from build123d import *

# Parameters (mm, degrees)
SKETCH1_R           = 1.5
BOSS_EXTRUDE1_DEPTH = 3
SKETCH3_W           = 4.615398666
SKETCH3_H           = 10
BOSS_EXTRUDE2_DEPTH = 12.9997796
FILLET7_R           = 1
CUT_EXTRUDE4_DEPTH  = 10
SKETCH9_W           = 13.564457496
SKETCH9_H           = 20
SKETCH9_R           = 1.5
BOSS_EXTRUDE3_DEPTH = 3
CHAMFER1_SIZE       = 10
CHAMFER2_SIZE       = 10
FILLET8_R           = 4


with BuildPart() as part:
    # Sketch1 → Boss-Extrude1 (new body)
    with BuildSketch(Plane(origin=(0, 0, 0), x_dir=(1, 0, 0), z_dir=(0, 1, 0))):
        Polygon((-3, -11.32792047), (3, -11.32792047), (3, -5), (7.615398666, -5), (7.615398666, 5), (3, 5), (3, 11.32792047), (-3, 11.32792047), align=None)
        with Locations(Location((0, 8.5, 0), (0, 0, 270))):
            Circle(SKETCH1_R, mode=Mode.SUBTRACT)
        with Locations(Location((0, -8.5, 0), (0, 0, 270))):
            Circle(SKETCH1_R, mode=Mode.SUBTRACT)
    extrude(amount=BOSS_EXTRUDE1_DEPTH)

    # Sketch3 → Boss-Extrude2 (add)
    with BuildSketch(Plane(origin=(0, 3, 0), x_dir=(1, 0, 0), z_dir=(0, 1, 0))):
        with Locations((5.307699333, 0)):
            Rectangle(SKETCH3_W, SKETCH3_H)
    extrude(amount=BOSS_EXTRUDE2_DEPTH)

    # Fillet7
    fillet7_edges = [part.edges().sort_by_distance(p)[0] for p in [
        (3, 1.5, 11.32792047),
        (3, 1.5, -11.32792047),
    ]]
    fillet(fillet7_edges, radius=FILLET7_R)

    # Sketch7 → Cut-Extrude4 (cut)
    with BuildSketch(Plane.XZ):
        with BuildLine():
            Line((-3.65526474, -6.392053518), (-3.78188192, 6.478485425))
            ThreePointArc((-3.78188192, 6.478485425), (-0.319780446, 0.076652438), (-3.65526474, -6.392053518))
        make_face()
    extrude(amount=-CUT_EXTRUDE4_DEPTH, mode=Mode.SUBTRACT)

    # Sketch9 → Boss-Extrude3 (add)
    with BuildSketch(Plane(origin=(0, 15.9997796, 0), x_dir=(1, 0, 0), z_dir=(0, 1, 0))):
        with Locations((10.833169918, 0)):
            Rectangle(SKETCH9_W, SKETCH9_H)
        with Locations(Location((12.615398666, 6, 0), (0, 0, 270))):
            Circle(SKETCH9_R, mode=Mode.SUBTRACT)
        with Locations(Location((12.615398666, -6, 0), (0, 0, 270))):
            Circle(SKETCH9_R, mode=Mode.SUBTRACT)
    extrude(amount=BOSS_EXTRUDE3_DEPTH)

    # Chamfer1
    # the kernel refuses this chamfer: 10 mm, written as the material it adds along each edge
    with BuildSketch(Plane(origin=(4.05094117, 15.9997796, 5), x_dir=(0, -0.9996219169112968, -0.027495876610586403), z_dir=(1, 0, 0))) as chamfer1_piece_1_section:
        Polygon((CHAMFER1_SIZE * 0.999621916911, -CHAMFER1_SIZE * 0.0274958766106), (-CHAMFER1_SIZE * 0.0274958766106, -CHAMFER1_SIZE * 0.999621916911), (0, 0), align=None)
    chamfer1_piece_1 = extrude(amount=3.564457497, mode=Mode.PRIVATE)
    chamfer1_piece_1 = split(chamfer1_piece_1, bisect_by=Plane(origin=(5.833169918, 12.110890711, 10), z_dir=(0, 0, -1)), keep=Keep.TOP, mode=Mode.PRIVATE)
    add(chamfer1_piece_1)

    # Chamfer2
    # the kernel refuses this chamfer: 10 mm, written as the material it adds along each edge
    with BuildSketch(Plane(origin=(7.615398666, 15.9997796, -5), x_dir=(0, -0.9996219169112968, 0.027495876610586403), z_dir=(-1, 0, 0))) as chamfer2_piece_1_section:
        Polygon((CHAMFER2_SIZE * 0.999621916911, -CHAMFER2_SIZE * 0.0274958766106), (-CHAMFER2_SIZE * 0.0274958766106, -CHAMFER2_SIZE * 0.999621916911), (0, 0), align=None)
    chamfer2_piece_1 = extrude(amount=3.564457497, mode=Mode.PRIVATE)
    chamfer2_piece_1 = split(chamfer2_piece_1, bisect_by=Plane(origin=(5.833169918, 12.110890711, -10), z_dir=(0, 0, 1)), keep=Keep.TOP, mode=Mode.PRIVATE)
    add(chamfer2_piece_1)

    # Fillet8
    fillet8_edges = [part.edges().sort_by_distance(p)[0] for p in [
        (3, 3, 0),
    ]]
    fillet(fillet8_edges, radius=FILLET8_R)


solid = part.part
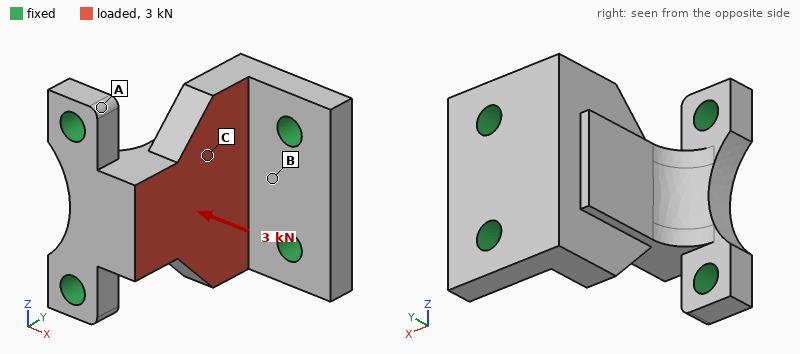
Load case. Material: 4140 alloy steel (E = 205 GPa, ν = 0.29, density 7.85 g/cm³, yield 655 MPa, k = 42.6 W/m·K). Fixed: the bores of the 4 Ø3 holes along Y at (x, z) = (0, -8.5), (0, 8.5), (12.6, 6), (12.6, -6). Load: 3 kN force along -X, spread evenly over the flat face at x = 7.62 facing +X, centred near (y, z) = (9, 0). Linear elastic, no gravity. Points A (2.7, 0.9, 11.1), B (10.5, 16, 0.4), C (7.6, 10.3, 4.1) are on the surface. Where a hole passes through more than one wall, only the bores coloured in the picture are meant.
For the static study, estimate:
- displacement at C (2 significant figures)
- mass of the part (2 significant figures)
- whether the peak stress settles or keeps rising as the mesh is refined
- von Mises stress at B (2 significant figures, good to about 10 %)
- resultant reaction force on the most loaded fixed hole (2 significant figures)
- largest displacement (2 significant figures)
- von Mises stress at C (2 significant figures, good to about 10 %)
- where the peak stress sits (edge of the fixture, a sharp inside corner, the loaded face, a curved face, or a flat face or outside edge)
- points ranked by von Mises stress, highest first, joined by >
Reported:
9.6 µm
17 g
keeps rising
57 MPa
820 N
13 µm
95 MPa
edge of the fixture
C > B > A
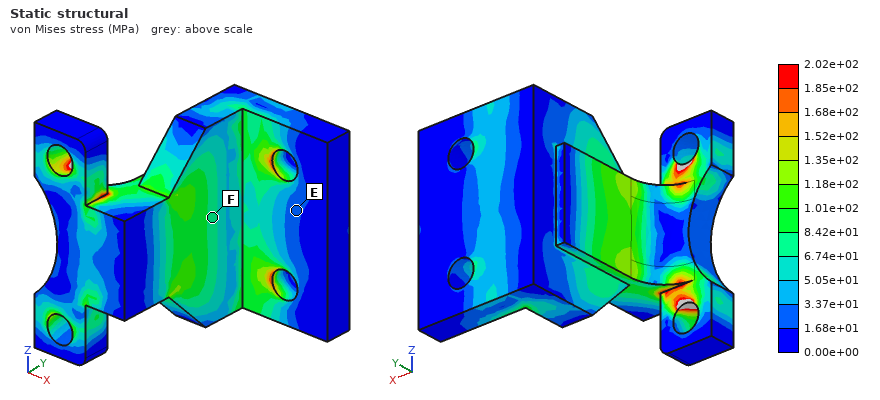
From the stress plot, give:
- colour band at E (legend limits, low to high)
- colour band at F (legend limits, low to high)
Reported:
1.68e+01 to 3.37e+01 MPa
6.74e+01 to 8.42e+01 MPa
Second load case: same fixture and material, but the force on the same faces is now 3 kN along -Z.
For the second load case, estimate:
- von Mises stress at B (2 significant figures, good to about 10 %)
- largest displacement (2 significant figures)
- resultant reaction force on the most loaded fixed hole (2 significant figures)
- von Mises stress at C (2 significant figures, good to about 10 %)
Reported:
50 MPa
8.5 µm
1.1 kN
45 MPa
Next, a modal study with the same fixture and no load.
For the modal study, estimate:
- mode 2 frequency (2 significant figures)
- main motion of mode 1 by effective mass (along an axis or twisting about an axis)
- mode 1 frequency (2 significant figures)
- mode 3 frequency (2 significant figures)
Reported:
42 kHz
along Y
23 kHz
44 kHz
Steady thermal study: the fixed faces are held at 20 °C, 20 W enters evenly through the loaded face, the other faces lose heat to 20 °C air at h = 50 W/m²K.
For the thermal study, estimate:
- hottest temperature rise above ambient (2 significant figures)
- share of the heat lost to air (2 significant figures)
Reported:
45 K
6.3 %
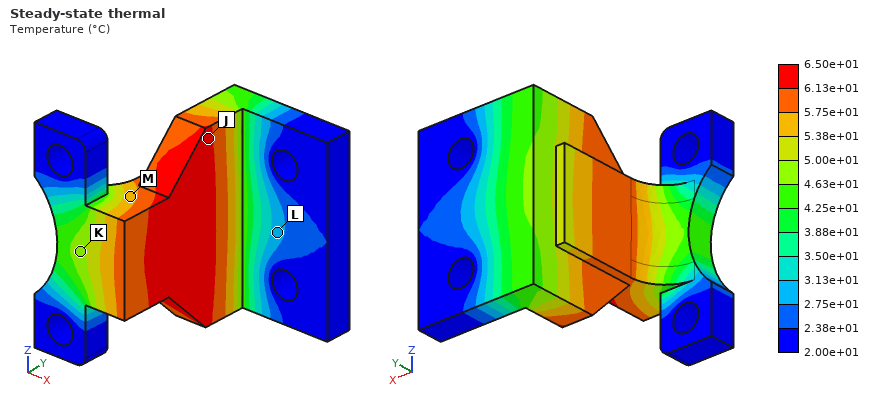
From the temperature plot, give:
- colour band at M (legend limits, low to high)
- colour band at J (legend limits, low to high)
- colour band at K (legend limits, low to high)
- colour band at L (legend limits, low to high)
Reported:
5.38e+01 to 5.75e+01 °C
6.13e+01 to 6.50e+01 °C
4.63e+01 to 5.00e+01 °C
2.75e+01 to 3.13e+01 °C
